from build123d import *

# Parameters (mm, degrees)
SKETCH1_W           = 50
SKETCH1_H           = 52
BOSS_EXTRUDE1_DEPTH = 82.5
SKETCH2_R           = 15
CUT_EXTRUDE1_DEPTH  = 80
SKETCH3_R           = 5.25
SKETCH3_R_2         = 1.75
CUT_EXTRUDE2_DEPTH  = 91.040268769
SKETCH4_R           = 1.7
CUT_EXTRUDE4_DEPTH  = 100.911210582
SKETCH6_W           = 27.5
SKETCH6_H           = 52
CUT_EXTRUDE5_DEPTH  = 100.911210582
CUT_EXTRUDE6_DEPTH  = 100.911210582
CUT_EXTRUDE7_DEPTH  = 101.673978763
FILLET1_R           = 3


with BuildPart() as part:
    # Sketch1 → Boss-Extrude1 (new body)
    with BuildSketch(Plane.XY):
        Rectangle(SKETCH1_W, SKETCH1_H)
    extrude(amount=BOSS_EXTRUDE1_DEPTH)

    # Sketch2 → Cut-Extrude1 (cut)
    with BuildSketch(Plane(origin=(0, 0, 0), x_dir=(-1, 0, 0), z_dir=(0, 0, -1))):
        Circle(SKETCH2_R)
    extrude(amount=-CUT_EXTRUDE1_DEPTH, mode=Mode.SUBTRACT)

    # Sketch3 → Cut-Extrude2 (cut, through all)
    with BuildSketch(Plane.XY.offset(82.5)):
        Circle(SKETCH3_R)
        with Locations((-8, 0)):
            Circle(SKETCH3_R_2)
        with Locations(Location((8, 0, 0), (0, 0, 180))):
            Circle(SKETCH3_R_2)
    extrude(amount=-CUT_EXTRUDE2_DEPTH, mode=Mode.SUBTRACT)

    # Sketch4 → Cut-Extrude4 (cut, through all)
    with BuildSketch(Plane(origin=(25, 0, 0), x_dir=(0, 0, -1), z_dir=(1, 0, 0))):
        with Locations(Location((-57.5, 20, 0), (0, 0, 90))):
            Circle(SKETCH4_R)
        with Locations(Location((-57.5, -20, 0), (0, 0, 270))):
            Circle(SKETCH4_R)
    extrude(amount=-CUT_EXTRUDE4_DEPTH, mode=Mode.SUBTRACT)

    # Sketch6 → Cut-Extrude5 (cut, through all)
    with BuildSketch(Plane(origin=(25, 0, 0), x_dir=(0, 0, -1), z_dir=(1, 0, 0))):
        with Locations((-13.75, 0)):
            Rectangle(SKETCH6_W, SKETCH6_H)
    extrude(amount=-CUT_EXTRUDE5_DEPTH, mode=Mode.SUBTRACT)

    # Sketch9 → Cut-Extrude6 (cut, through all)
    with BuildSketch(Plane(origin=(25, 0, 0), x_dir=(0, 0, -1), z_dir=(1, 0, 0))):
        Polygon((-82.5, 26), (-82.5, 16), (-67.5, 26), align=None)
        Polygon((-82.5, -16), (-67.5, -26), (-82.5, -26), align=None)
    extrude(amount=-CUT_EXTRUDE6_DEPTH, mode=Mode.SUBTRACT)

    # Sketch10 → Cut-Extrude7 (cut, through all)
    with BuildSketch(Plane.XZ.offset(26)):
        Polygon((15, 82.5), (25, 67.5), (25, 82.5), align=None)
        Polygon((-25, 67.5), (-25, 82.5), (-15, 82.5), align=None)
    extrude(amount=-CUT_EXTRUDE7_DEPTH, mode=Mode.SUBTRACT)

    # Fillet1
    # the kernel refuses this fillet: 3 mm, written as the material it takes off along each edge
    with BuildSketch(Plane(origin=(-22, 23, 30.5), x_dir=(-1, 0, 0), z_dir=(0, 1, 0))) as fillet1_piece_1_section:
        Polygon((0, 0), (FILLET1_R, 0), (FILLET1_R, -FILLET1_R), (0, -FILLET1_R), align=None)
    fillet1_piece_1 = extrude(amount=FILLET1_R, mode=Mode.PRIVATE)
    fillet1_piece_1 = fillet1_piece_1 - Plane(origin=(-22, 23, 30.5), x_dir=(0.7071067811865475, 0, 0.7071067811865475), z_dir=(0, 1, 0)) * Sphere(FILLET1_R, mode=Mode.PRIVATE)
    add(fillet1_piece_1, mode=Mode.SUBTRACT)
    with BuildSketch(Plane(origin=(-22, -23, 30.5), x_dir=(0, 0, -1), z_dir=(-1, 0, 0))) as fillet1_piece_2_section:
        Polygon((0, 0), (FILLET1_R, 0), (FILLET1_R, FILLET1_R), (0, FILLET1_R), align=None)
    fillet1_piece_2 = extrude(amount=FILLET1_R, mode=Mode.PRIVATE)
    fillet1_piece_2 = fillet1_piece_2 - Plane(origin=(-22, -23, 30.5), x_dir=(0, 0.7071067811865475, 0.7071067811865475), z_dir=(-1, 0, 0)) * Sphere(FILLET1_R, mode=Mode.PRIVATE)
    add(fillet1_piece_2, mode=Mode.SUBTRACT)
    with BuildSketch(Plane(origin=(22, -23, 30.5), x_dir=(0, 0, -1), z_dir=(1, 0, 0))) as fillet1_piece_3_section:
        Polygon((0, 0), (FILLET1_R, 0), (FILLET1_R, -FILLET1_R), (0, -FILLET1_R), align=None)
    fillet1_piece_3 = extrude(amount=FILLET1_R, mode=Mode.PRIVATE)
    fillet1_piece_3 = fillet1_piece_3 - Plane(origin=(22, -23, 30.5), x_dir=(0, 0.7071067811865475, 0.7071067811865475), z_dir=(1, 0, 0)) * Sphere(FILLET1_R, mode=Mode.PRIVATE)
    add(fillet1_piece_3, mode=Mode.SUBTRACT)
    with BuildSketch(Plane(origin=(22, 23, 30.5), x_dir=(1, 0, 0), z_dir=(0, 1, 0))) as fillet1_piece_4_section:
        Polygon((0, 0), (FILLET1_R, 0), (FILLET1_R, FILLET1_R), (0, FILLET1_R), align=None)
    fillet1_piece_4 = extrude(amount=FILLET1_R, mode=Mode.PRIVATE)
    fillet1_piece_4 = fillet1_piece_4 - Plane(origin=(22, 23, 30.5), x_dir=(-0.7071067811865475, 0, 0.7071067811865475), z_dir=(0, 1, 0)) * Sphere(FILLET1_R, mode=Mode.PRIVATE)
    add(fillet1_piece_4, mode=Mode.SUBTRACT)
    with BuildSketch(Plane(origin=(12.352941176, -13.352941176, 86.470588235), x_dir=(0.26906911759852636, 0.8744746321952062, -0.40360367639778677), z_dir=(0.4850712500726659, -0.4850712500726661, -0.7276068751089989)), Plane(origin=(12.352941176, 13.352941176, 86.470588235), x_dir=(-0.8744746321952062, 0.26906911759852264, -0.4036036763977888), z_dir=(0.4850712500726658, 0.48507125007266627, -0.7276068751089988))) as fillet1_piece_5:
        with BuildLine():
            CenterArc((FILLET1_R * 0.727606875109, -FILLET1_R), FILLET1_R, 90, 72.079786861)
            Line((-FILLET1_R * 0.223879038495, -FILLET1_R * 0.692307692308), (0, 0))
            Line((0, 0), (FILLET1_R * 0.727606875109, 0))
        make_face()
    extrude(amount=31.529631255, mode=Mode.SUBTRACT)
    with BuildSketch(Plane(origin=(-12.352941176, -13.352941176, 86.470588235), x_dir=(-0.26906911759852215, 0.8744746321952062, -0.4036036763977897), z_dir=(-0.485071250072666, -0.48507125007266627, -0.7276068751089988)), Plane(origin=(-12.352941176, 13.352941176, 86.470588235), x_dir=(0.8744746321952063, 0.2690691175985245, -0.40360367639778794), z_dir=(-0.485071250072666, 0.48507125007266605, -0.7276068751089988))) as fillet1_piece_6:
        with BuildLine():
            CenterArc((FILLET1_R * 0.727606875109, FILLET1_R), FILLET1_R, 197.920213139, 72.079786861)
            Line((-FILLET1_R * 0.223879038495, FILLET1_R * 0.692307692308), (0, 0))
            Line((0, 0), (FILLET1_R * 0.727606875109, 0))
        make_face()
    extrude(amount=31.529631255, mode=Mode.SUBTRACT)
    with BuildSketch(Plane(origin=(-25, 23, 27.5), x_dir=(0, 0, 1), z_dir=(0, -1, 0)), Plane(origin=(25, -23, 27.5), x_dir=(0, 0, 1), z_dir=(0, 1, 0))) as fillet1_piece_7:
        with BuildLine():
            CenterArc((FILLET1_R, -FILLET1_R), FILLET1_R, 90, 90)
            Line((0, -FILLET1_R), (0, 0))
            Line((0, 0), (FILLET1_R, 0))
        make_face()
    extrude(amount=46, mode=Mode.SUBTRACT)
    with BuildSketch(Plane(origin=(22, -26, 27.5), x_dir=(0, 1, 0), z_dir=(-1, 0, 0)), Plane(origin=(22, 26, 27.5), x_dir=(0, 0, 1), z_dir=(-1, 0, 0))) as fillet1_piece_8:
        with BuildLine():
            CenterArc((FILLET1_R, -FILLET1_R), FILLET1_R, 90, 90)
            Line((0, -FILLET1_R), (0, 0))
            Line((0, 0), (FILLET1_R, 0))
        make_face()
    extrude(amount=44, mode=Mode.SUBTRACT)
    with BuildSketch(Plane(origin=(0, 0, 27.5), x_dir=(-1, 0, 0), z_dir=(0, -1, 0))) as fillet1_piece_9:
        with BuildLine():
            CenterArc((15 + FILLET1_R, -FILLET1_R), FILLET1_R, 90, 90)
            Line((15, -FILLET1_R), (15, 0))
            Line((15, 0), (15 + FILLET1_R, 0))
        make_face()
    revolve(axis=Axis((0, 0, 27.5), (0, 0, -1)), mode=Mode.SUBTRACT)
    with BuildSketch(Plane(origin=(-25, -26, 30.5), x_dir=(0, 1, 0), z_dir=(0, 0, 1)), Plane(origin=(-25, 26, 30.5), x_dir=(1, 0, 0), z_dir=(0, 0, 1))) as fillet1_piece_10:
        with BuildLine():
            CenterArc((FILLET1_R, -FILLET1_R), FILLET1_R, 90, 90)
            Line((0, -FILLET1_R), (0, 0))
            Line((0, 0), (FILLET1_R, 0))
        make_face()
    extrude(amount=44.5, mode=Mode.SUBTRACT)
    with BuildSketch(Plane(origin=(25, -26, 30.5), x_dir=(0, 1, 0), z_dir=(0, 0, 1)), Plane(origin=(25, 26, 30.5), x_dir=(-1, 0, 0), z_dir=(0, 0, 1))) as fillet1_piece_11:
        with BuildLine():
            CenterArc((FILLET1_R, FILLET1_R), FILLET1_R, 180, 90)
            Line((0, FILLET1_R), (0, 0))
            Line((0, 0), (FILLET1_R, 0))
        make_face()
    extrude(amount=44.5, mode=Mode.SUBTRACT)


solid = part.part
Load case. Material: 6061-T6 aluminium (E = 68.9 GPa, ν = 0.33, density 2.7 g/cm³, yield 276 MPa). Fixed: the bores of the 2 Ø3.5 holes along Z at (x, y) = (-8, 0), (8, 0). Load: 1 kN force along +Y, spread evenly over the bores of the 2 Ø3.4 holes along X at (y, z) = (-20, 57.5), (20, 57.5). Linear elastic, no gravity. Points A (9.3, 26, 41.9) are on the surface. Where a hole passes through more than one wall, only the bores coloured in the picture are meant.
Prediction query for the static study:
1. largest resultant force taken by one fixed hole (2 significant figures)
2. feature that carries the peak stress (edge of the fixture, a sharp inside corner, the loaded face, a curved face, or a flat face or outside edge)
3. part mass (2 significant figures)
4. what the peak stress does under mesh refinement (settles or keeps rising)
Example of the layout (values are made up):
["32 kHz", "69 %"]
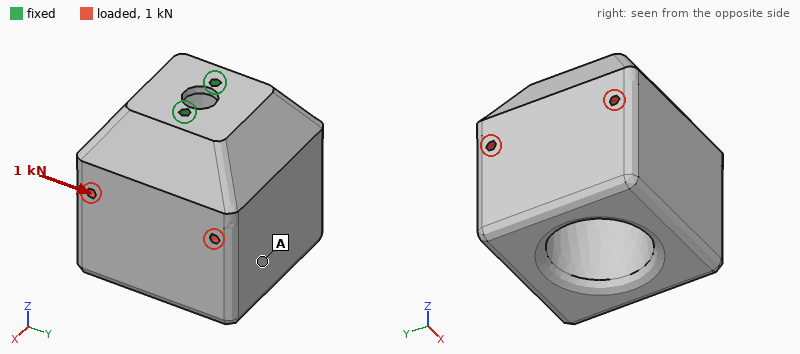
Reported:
["510 N", "edge of the fixture", "240 g", "keeps rising"]
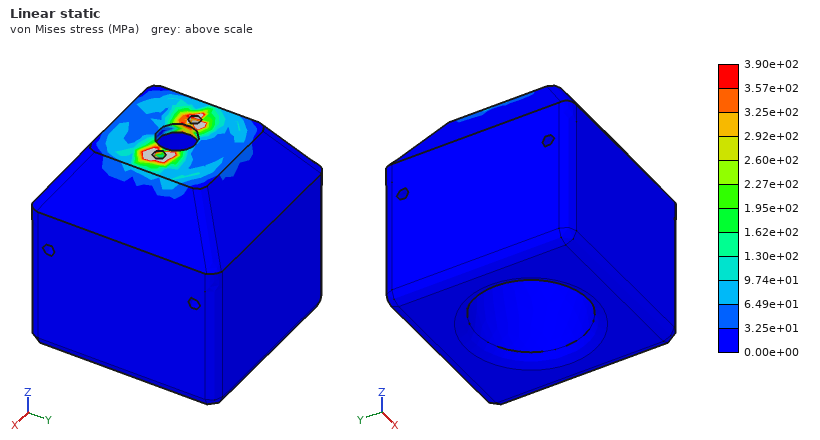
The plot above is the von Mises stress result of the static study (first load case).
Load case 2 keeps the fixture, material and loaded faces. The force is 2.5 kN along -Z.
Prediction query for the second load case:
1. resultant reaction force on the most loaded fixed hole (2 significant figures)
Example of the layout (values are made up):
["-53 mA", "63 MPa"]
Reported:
["1.3 kN"]
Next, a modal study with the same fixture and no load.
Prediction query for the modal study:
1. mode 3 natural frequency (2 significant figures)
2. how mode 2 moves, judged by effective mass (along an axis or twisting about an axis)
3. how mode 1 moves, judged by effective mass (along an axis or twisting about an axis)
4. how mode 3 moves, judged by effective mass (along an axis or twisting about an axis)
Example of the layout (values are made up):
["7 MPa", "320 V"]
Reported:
["2600 Hz", "along X", "along Y", "twisting about Z"]
